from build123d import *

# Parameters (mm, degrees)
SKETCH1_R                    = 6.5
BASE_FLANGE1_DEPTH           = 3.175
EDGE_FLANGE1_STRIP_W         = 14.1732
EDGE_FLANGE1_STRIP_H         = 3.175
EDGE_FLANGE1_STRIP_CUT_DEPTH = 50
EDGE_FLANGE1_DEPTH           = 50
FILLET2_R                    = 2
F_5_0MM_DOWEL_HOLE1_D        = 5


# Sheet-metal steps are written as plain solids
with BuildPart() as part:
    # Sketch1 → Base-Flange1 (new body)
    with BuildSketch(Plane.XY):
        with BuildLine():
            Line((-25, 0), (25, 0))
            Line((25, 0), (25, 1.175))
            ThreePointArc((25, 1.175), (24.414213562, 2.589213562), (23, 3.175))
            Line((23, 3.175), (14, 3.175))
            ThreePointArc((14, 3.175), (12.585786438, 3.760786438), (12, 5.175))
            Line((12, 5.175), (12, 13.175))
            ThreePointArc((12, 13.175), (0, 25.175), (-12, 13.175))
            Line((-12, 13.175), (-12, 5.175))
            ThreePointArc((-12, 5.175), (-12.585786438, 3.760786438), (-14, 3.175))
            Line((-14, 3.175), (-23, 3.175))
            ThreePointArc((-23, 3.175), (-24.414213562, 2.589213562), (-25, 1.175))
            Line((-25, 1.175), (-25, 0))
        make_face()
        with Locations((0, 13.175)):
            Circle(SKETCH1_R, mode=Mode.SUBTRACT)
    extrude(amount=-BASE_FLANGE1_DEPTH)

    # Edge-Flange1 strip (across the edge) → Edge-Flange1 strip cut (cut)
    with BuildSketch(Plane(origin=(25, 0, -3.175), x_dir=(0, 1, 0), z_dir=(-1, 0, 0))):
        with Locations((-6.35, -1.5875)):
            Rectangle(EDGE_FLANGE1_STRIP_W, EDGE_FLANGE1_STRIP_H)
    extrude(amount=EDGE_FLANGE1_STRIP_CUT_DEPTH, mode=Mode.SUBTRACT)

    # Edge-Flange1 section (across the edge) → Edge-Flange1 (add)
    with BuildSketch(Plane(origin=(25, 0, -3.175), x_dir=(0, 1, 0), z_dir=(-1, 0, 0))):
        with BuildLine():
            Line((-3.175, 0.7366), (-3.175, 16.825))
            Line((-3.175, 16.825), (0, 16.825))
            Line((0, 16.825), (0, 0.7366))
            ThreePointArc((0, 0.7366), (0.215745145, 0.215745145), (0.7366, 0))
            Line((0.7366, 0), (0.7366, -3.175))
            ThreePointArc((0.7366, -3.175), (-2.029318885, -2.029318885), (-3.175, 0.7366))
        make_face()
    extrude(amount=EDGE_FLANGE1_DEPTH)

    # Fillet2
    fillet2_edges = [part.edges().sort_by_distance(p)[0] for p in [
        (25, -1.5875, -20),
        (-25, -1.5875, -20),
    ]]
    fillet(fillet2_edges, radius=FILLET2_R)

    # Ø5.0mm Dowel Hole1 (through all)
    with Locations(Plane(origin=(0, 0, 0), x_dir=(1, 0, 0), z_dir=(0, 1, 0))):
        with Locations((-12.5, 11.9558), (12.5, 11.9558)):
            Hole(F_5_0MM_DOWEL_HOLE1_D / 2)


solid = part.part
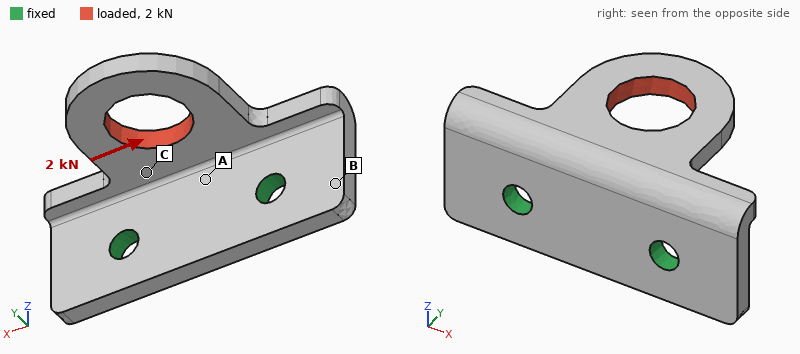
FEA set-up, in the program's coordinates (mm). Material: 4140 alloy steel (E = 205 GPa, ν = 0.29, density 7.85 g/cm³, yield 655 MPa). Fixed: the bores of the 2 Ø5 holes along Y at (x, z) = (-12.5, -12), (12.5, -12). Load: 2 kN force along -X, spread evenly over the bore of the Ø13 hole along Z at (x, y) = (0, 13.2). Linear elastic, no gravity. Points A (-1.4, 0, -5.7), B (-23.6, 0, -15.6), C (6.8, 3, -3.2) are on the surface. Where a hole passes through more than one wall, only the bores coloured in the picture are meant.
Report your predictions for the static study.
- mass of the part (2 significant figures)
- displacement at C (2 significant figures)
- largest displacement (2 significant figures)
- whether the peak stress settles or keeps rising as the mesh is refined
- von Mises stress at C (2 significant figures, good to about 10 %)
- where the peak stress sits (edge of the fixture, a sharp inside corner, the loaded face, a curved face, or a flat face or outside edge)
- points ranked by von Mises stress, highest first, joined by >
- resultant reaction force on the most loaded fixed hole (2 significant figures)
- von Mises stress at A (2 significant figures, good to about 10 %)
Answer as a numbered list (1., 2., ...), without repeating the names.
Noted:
1. 35 g
2. 16 µm
3. 70 µm
4. keeps rising
5. 77 MPa
6. edge of the fixture
7. A > C > B
8. 1.6 kN
9. 110 MPa
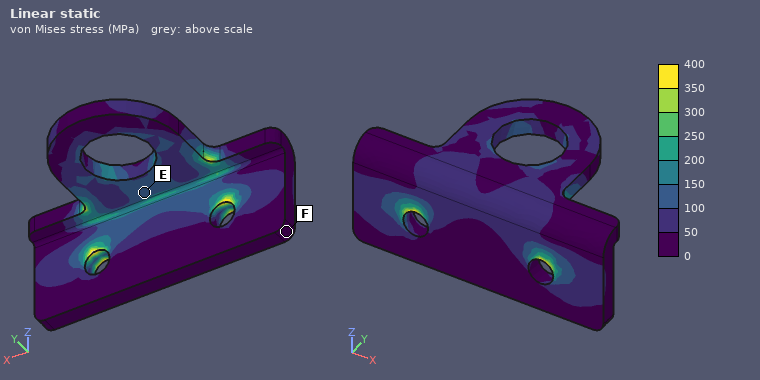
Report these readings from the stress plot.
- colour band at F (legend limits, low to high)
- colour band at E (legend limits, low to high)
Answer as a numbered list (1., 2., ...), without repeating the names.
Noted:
1. 0 to 50 MPa
2. 100 to 150 MPa
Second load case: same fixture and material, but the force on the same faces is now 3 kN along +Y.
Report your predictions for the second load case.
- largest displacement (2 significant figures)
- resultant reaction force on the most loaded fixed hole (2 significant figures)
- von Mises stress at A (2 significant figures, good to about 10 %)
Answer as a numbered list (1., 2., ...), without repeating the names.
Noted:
1. 0.17 mm
2. 1.5 kN
3. 110 MPa
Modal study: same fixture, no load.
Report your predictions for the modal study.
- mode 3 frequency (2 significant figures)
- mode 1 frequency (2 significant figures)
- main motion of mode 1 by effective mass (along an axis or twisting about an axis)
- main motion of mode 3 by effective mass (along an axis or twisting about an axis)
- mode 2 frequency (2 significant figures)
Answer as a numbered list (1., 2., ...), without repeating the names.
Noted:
1. 11 kHz
2. 3500 Hz
3. along Z
4. along Y
5. 8700 Hz
